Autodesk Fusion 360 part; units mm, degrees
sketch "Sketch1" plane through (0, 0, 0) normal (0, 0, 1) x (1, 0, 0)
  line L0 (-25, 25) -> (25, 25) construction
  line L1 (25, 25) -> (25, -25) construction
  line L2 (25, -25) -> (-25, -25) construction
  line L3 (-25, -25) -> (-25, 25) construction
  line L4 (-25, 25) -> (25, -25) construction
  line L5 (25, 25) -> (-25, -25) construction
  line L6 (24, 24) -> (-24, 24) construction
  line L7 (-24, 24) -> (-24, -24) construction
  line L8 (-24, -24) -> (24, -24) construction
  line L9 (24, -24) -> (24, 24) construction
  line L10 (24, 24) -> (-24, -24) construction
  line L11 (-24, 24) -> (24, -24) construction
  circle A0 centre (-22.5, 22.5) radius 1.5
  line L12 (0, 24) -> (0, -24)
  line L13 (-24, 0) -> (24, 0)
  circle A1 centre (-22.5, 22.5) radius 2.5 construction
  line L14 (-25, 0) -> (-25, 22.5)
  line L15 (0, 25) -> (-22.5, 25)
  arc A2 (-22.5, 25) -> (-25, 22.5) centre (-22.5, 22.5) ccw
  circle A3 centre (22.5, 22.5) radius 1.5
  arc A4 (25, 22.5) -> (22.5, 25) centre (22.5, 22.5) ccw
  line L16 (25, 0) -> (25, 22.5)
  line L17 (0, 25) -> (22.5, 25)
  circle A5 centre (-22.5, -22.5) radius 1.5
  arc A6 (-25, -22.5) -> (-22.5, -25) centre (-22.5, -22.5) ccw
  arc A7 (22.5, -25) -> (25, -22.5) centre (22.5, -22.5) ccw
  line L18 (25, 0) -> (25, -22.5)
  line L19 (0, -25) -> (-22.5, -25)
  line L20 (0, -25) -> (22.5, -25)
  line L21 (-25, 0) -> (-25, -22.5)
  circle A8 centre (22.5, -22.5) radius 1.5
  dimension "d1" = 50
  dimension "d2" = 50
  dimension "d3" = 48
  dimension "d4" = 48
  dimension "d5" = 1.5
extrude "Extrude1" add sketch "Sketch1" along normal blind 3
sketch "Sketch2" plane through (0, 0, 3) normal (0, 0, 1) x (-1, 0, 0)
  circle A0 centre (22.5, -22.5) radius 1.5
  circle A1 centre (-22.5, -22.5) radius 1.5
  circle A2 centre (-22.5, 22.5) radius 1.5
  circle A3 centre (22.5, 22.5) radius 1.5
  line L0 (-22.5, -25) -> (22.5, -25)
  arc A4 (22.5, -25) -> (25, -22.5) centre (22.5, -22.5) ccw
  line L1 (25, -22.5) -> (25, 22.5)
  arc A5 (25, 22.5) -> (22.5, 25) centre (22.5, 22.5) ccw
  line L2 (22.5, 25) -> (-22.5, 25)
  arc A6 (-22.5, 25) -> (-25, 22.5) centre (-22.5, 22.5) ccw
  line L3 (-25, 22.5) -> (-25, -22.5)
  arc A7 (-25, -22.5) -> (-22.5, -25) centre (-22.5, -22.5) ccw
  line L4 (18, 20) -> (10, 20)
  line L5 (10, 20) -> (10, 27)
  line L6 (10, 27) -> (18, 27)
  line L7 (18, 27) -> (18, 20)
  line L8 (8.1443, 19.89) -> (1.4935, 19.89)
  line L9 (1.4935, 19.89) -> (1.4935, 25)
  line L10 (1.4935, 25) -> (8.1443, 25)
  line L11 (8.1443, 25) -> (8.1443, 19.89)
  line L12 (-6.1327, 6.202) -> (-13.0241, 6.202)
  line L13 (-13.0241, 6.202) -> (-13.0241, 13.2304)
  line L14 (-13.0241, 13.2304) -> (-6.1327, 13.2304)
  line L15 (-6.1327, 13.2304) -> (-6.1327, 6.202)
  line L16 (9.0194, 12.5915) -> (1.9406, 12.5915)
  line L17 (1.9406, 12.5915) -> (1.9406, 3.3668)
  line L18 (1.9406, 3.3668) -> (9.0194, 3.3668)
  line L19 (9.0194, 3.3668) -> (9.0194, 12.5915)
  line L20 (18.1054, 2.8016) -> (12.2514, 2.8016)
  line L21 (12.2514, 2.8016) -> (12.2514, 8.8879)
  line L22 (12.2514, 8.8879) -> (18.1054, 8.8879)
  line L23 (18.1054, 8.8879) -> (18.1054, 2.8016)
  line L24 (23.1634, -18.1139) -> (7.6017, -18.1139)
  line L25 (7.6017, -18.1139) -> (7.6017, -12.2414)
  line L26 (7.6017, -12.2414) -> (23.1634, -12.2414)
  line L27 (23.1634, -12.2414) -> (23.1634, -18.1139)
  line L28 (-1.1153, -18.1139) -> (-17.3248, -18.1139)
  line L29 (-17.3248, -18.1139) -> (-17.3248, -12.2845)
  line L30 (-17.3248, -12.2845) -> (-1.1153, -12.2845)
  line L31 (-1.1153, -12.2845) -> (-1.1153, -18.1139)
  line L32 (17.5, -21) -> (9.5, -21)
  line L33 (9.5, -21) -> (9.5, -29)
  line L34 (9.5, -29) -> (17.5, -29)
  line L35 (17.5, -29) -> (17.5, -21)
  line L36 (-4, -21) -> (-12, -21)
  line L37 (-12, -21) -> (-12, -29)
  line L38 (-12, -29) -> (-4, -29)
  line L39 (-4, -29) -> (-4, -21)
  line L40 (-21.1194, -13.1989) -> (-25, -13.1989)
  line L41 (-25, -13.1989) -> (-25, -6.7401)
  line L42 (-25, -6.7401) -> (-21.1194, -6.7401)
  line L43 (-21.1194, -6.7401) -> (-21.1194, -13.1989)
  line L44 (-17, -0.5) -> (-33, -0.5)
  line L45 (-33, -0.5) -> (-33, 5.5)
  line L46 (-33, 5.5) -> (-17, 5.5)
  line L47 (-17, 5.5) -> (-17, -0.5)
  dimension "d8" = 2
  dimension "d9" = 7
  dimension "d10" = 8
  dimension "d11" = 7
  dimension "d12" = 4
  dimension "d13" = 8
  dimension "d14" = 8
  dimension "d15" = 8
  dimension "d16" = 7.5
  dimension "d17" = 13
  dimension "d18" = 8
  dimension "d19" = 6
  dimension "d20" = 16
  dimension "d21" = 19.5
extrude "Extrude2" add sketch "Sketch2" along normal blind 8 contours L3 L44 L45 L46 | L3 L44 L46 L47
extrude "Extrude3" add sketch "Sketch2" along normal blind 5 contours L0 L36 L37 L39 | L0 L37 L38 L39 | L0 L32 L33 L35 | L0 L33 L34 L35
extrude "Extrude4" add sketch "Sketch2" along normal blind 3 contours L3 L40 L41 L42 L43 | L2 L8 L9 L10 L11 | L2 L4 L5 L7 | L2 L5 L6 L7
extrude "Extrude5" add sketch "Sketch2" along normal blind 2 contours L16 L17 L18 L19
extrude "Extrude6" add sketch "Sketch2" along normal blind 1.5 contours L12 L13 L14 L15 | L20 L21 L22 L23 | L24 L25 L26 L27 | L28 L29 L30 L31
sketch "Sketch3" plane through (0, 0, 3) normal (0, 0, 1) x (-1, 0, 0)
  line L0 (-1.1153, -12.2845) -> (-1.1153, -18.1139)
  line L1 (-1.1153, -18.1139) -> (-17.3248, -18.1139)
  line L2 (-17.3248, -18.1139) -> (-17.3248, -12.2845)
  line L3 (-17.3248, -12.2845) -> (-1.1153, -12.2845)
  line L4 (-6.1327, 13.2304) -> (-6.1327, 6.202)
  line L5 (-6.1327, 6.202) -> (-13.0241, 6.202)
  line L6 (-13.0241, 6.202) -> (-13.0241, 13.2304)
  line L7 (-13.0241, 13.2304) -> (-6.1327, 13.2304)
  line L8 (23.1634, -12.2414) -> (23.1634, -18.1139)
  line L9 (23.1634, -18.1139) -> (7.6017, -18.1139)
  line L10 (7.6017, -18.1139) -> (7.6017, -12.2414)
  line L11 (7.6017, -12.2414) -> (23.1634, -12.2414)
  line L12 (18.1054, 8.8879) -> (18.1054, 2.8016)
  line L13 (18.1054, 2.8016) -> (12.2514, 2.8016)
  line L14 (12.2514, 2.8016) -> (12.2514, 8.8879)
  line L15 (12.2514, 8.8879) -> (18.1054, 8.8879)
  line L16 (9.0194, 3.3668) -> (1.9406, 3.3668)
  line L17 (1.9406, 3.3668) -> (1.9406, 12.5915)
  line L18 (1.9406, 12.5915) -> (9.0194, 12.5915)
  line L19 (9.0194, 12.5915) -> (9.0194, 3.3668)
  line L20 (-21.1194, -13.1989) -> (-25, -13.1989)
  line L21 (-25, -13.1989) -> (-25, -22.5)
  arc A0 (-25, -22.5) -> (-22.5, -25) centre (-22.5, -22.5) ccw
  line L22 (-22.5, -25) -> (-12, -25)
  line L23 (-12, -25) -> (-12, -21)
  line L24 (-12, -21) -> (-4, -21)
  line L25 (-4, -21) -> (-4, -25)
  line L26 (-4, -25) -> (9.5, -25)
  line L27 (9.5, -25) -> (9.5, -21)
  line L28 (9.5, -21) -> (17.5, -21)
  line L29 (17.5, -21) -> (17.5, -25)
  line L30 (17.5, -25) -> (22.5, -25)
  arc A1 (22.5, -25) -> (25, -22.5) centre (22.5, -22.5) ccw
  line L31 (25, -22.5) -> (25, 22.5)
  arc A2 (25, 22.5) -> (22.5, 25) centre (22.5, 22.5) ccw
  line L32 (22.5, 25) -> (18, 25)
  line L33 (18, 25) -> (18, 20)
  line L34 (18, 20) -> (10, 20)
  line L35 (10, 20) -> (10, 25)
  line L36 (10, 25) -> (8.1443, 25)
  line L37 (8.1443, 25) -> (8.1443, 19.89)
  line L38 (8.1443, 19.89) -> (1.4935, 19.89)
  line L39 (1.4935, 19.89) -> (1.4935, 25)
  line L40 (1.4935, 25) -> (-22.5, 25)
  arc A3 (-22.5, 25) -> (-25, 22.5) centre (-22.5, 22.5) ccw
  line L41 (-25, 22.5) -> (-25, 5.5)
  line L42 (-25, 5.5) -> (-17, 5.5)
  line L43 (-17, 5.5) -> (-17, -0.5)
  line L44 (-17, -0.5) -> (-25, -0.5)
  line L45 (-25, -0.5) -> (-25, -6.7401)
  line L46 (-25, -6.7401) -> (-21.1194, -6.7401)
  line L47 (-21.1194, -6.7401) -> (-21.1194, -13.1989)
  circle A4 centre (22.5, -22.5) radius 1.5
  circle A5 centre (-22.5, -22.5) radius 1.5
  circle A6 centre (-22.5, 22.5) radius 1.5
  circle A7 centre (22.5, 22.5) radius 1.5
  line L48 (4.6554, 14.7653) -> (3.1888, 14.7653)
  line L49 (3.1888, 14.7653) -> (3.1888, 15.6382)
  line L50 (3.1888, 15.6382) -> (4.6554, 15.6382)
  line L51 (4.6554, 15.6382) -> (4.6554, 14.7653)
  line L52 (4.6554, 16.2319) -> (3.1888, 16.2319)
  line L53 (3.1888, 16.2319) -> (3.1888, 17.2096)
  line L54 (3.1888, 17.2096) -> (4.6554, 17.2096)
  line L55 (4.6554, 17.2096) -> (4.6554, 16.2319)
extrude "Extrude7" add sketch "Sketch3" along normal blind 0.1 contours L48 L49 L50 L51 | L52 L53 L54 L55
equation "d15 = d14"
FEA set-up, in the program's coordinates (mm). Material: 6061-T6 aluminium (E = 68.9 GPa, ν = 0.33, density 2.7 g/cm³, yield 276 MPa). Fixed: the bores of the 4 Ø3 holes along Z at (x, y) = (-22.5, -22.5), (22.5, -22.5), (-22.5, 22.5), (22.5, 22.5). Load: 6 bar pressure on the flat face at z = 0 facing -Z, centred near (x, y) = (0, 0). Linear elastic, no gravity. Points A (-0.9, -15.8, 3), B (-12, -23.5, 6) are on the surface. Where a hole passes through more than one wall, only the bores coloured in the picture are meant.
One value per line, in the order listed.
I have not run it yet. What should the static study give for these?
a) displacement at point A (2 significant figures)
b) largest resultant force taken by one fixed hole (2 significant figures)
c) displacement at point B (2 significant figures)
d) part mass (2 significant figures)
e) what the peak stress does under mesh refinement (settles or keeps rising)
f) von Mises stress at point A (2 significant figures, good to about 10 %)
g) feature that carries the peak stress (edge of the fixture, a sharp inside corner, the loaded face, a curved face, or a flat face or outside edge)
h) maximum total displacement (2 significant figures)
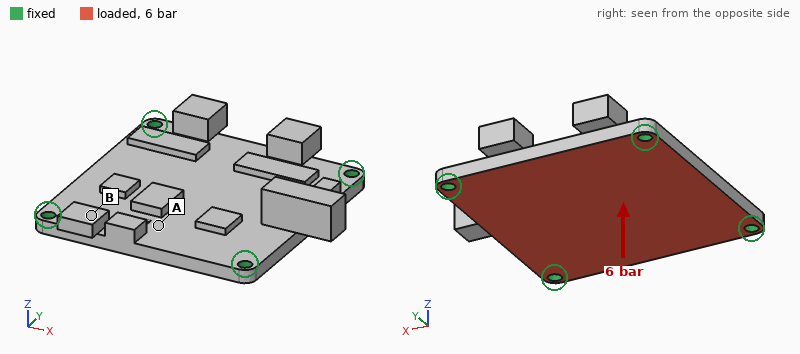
0.078 mm
380 N
0.036 mm
26 g
keeps rising
39 MPa
edge of the fixture
0.11 mm
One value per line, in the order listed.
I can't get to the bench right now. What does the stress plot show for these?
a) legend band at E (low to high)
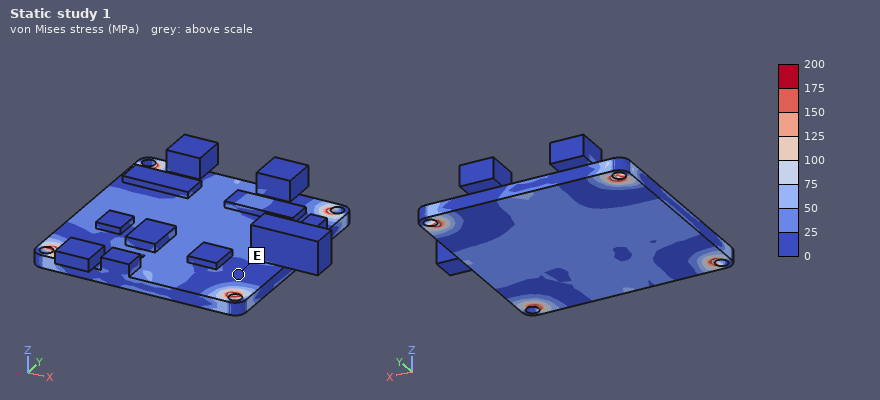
0 to 25 MPa
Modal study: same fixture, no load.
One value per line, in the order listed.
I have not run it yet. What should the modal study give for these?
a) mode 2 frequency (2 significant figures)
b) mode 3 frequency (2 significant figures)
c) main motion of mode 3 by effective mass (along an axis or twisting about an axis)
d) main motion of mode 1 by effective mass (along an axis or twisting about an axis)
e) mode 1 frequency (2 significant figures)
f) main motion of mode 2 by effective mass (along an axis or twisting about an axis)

5500 Hz
7600 Hz
twisting about X
along Z
4600 Hz
twisting about Y
